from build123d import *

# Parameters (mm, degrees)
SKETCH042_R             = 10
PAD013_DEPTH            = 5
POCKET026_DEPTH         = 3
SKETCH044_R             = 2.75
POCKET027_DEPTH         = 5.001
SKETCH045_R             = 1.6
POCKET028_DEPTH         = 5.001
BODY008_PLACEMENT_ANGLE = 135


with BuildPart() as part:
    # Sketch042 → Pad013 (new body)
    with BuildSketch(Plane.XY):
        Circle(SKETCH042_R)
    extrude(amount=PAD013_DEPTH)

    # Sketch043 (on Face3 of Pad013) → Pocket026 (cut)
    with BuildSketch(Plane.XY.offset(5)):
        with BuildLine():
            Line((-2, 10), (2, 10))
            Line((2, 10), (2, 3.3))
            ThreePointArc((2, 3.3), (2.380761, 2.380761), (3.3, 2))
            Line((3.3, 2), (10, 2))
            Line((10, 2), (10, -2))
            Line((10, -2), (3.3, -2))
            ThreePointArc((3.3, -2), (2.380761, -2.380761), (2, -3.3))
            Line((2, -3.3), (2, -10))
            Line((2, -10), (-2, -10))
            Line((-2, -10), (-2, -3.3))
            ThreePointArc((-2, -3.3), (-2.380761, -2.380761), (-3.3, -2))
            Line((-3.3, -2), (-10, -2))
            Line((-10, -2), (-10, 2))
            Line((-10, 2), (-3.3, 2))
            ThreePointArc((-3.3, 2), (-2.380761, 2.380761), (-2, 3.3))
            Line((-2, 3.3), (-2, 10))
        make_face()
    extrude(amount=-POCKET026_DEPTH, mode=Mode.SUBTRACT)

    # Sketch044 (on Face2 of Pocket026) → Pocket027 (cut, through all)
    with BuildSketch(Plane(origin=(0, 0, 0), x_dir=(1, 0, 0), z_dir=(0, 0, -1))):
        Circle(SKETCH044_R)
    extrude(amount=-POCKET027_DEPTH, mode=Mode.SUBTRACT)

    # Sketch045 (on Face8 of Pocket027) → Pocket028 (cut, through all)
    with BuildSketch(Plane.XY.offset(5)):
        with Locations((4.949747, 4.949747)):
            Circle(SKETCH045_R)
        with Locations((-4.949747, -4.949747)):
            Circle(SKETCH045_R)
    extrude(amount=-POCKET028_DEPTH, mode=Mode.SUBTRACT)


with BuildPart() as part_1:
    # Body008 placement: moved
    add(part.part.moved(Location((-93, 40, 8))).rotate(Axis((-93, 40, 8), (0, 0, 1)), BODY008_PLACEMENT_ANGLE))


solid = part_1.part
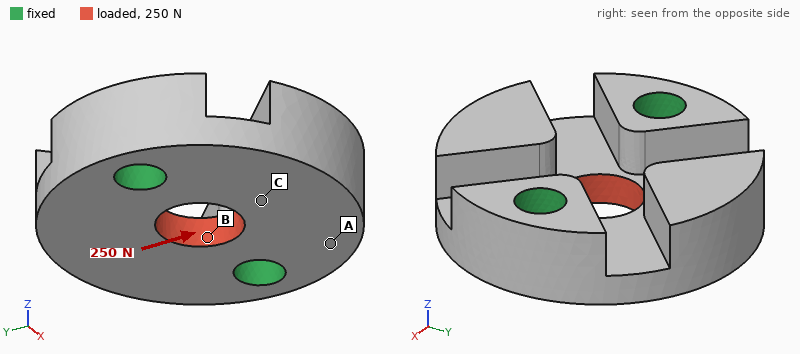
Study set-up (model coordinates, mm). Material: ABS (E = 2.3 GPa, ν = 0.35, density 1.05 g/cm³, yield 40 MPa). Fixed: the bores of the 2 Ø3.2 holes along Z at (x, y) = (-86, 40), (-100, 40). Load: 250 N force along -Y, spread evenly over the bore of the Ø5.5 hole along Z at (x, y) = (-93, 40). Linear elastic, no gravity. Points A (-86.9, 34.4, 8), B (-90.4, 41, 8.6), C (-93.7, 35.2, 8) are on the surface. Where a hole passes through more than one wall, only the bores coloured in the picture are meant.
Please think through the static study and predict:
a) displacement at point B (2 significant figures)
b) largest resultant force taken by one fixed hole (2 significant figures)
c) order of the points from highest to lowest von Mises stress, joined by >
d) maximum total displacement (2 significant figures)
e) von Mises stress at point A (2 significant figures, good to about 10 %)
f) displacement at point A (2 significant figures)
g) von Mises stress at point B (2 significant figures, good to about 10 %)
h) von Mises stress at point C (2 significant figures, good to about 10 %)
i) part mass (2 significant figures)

24 µm
130 N
B > C > A
29 µm
2.8 MPa
10 µm
12 MPa
6.4 MPa
1.1 g
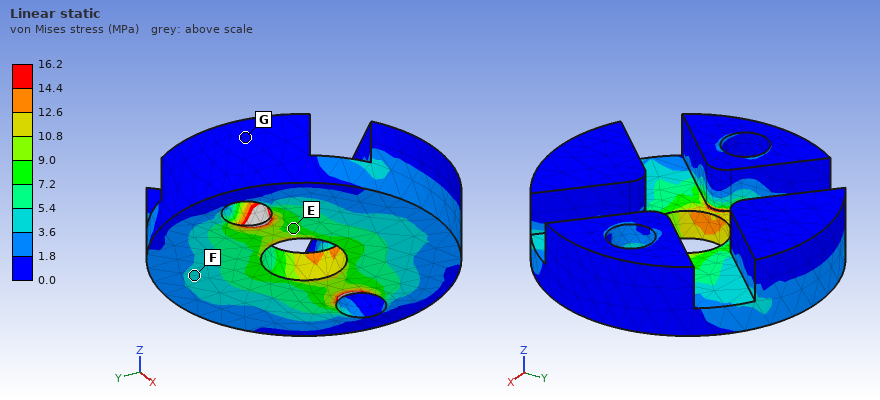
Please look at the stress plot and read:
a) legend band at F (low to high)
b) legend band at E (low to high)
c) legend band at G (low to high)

3.6 to 5.4 MPa
7.2 to 9.0 MPa
0.0 to 1.8 MPa
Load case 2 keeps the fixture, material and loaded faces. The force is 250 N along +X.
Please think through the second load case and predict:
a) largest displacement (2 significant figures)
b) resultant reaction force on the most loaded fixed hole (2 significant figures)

22 µm
130 N
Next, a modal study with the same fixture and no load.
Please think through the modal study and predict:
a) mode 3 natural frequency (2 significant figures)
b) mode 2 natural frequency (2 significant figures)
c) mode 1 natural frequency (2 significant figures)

14 kHz
5500 Hz
5500 Hz
